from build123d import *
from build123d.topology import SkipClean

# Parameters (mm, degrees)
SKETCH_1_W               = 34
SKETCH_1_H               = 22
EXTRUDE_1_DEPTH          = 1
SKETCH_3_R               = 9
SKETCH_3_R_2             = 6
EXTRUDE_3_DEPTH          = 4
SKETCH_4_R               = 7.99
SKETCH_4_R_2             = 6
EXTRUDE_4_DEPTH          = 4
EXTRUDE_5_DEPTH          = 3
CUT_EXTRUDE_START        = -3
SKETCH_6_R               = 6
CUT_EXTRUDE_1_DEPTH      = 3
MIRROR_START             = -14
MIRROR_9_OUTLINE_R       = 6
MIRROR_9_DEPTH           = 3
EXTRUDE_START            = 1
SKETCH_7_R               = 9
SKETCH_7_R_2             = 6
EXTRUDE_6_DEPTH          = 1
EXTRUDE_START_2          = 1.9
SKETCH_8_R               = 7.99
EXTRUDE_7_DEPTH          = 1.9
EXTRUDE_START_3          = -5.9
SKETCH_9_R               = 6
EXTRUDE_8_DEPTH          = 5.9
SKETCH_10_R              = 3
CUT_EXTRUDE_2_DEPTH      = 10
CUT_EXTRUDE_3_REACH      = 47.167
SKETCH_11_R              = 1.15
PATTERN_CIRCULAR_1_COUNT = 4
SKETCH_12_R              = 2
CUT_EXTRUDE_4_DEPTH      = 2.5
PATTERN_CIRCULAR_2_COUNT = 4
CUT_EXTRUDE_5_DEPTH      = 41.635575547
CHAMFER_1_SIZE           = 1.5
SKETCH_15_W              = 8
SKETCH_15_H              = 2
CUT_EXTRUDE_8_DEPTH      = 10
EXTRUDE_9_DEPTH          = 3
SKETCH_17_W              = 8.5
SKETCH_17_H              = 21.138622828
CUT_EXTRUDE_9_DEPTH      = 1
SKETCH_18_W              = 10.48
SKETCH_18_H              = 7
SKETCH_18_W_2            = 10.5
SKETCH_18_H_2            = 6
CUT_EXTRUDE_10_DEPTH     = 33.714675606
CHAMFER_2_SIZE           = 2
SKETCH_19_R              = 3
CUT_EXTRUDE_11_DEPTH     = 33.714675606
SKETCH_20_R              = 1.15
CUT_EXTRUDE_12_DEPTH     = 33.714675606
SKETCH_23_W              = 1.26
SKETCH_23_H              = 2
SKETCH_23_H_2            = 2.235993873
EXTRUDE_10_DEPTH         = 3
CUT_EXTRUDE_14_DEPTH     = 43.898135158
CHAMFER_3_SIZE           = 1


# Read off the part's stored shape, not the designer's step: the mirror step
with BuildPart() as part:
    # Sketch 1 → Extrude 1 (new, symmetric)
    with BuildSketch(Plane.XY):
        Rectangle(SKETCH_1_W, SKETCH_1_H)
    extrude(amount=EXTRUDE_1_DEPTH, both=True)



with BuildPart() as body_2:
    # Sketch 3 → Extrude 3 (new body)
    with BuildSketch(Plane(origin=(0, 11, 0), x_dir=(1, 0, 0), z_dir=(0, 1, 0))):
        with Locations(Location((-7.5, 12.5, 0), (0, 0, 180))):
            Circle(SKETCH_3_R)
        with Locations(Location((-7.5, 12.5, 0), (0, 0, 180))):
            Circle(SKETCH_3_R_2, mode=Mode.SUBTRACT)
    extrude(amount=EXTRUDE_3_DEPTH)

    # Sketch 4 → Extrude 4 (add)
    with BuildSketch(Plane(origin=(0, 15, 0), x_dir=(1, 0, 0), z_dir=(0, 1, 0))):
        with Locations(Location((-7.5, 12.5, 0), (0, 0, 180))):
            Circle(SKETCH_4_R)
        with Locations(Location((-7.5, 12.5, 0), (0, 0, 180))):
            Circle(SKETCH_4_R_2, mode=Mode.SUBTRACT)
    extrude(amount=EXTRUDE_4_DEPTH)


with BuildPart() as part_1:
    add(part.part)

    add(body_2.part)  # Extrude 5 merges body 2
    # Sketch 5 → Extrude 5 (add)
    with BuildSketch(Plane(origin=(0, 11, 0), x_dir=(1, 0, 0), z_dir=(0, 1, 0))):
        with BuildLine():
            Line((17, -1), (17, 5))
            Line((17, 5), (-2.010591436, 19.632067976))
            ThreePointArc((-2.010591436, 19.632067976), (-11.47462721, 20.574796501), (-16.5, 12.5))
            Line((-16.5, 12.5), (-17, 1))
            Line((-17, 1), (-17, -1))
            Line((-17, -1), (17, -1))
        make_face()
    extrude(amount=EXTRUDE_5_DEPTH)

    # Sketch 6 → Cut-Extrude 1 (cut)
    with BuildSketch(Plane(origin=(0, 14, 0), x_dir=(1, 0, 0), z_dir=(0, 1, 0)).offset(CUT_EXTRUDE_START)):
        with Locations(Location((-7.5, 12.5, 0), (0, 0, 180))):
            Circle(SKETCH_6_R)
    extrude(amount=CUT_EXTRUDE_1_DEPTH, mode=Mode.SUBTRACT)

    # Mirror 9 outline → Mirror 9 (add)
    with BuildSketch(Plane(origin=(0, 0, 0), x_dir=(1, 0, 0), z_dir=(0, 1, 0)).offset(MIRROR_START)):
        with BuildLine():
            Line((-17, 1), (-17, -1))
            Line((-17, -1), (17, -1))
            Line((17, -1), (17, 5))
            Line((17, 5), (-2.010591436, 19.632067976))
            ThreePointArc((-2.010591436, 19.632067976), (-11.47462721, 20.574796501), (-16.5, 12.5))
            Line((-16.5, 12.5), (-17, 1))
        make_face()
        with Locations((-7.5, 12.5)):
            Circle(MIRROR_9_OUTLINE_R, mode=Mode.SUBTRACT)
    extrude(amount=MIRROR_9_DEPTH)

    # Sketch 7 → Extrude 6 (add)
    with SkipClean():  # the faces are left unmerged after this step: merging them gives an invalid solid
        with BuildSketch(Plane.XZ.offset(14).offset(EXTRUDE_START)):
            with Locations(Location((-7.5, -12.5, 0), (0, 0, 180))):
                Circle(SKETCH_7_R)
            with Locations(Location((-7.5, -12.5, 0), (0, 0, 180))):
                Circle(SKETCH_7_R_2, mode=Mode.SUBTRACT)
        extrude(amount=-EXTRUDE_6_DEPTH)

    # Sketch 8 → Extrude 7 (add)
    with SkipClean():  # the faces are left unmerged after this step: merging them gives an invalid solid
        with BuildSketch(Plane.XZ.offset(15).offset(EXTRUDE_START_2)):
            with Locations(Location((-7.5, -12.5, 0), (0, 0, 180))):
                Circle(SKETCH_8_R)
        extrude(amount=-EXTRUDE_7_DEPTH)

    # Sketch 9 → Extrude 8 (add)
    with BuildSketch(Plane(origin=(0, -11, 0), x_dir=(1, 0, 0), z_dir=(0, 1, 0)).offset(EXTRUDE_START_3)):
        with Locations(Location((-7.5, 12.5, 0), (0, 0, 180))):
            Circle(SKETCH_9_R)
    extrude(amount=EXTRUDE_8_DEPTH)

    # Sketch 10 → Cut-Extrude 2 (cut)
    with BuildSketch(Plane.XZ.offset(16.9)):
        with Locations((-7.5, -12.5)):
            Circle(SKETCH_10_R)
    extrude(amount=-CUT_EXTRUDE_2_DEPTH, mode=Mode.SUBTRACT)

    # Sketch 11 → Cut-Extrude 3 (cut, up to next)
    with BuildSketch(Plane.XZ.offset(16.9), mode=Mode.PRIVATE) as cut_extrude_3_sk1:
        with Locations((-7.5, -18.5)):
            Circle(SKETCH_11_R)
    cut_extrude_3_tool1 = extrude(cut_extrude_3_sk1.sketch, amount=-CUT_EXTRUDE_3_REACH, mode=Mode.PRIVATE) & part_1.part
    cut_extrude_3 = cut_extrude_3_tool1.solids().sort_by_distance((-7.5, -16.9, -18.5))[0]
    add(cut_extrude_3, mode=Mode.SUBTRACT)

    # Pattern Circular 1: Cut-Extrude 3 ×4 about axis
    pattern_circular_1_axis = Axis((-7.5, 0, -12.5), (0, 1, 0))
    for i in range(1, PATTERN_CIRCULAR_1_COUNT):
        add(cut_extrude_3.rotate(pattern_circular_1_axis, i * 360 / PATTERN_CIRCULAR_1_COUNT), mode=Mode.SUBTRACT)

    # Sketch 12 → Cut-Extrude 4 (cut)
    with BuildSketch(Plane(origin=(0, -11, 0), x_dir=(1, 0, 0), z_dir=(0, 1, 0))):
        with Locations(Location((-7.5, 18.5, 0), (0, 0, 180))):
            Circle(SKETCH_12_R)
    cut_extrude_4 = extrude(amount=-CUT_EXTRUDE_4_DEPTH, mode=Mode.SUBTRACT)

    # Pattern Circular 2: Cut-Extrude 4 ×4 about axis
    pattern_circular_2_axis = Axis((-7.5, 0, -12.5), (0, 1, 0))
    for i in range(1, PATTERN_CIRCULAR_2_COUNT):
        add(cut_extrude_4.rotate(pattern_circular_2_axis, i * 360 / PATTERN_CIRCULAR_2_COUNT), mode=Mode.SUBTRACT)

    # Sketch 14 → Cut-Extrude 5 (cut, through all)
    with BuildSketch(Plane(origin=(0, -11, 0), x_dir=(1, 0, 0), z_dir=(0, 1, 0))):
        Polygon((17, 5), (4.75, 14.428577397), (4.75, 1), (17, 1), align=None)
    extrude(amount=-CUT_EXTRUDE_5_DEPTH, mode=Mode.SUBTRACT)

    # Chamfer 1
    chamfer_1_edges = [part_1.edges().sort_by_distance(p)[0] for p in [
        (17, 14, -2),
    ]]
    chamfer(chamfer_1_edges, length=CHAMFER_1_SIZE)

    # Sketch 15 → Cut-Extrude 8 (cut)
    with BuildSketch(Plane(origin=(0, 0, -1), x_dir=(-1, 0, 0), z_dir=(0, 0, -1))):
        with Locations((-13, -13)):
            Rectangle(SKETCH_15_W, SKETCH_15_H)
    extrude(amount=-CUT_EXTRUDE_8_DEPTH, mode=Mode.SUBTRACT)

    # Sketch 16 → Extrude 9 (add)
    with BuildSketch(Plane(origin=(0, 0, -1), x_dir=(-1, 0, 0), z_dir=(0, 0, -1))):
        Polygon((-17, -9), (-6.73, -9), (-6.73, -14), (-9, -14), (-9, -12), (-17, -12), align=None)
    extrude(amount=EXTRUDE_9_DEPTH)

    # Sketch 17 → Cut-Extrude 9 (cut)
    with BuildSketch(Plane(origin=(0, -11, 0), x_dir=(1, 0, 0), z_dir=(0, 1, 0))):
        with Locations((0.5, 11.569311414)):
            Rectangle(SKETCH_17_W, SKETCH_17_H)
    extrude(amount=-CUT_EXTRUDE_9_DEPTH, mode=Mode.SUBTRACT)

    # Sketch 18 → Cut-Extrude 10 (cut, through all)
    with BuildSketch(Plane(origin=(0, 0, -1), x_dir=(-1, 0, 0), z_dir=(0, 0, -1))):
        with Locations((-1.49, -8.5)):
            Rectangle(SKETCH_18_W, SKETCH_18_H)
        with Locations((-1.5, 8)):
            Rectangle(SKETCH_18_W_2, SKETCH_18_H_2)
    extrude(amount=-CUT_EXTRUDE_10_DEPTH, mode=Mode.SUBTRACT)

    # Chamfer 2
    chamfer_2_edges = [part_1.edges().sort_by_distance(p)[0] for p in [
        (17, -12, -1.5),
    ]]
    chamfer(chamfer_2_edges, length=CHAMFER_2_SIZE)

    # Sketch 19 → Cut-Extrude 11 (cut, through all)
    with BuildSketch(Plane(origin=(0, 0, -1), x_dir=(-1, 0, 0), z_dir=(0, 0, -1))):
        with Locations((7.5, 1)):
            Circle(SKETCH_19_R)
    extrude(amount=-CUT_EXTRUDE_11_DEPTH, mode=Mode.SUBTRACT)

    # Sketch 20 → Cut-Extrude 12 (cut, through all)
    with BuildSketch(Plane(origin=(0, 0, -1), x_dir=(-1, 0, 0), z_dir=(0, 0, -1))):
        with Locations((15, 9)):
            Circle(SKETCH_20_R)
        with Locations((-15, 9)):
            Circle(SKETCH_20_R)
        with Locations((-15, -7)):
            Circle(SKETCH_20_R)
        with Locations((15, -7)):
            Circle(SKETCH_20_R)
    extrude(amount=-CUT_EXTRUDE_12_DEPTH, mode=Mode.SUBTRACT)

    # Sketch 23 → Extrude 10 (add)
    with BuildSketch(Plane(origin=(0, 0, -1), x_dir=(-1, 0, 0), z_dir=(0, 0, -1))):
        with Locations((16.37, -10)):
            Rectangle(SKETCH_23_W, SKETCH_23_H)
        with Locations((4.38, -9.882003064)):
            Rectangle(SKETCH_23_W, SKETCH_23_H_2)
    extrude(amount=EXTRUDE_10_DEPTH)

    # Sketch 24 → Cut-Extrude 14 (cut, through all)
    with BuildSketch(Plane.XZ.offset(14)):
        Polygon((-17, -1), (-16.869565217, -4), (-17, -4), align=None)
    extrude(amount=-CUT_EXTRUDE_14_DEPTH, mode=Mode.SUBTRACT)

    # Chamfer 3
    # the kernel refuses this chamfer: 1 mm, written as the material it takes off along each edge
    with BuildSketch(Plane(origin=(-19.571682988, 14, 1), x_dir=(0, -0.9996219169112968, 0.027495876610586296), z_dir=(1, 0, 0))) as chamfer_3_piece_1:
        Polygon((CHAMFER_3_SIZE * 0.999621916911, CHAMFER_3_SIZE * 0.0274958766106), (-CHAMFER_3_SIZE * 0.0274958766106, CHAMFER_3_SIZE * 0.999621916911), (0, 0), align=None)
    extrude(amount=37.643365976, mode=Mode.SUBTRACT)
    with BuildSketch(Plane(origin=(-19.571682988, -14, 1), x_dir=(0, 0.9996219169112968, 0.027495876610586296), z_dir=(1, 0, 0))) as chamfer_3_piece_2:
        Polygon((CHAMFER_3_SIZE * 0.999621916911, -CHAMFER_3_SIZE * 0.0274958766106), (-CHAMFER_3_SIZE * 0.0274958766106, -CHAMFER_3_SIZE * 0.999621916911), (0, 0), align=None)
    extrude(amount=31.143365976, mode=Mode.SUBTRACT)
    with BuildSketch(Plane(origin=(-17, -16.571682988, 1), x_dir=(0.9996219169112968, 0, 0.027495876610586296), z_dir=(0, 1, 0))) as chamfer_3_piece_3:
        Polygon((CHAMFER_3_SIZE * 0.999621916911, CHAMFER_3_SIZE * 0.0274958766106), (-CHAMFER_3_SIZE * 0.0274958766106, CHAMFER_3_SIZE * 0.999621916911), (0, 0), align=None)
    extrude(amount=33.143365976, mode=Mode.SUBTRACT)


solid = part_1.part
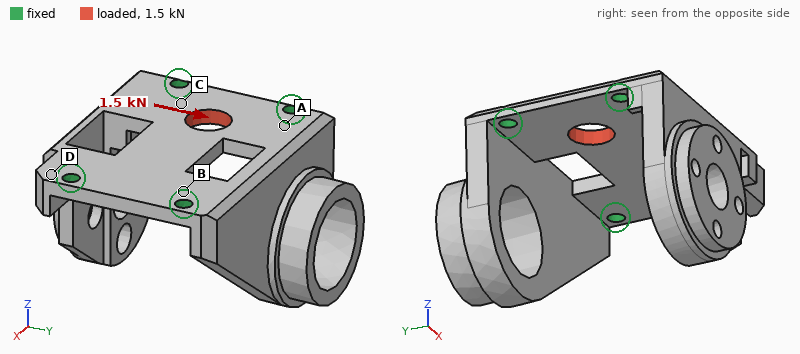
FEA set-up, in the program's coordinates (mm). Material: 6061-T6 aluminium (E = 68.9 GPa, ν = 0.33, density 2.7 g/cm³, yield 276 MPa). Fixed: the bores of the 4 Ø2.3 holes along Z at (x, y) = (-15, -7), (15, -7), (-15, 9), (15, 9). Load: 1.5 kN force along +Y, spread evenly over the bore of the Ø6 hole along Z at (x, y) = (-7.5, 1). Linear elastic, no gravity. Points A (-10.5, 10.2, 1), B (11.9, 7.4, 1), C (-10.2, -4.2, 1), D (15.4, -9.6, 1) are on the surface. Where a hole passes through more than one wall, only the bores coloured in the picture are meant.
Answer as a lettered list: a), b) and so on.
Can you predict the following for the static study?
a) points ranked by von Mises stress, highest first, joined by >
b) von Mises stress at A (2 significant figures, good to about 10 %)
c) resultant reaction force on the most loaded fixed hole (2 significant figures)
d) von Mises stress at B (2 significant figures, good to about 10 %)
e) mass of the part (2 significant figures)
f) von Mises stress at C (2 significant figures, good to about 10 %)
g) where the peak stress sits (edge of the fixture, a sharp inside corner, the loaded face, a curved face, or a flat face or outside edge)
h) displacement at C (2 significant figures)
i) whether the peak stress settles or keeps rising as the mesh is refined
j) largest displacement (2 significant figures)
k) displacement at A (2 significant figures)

a) C > A > B > D
b) 29 MPa
c) 660 N
d) 18 MPa
e) 12 g
f) 42 MPa
g) edge of the fixture
h) 6.4 µm
i) keeps rising
j) 18 µm
k) 6.3 µm
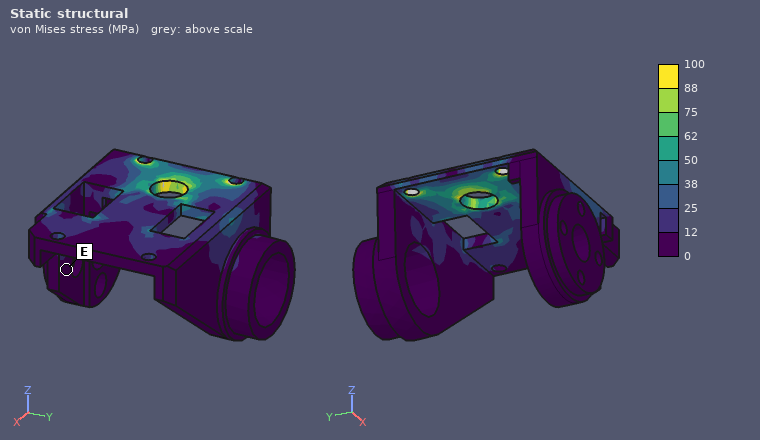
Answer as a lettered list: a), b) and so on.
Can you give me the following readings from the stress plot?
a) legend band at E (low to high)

a) 0 to 12 MPa
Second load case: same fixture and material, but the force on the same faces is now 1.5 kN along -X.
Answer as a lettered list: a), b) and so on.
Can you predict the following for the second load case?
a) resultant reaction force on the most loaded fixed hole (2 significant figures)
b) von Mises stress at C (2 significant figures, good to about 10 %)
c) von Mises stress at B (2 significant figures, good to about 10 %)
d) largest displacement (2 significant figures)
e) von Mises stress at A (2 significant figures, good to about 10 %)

a) 600 N
b) 37 MPa
c) 20 MPa
d) 9.3 µm
e) 15 MPa
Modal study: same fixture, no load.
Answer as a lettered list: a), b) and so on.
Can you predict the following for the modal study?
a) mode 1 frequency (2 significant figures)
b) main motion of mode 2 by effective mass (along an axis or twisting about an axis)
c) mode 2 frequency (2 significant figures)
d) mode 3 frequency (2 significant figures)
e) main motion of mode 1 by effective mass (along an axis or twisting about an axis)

a) 2400 Hz
b) along Y
c) 3200 Hz
d) 5000 Hz
e) along Y
